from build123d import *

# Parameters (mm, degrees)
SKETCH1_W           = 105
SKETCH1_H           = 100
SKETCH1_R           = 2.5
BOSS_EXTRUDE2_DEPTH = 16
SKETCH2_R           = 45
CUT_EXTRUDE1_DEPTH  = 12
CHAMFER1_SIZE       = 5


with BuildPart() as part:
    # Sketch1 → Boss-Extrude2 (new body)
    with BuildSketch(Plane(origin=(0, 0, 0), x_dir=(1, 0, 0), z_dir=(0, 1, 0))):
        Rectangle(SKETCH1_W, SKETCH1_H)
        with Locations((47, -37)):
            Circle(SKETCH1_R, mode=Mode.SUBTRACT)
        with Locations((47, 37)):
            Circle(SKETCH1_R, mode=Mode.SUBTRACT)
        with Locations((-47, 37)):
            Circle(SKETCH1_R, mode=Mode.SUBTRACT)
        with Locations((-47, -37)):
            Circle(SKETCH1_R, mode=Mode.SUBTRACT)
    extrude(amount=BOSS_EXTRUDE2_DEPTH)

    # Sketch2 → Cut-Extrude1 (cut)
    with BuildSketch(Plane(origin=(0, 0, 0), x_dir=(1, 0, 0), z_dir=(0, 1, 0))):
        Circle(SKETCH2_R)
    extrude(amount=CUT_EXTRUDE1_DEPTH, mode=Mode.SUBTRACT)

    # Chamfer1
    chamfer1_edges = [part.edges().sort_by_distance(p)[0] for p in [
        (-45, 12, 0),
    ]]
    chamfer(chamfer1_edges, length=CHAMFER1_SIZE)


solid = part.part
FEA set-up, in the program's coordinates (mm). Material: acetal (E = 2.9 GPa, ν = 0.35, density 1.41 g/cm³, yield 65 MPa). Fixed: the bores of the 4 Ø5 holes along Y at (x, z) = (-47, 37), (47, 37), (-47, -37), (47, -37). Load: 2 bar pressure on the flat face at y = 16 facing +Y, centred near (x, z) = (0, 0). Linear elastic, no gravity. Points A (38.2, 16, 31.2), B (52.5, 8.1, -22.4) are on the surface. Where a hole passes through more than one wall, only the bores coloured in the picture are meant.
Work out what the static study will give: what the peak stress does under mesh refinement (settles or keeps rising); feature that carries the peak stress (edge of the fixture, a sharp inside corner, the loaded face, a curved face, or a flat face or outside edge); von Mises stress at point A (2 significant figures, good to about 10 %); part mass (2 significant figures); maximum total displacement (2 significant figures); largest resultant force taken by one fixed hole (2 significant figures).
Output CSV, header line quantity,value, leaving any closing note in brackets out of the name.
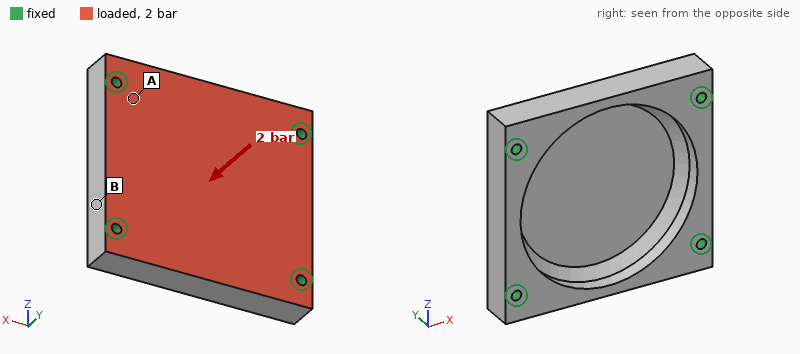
quantity,value
what the peak stress does under mesh refinement,keeps rising
feature that carries the peak stress,edge of the fixture
von Mises stress at point A,3.6 MPa
part mass,130 g
maximum total displacement,0.77 mm
largest resultant force taken by one fixed hole,600 N
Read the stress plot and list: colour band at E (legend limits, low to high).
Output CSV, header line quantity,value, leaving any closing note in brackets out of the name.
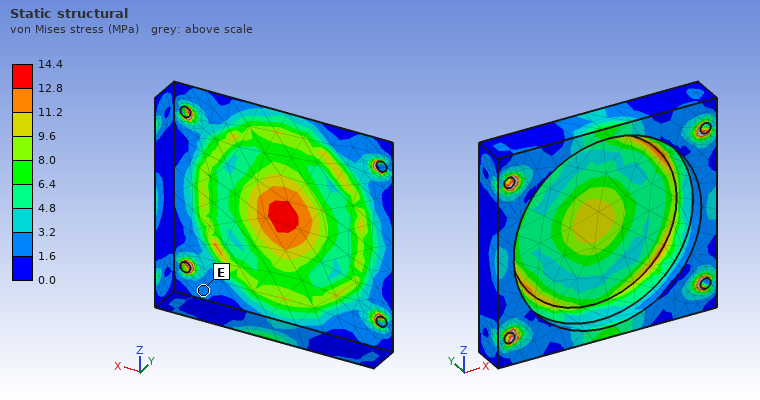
quantity,value
colour band at E,1.6 to 3.2 MPa
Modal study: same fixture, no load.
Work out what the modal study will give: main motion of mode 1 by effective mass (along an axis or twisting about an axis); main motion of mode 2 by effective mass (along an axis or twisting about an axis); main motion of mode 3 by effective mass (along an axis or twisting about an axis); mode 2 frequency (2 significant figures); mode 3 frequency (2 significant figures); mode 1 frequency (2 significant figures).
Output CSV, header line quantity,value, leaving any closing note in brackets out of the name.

quantity,value
main motion of mode 1 by effective mass,along Y
main motion of mode 2 by effective mass,twisting about X
main motion of mode 3 by effective mass,along Y
mode 2 frequency,2200 Hz
mode 3 frequency,2500 Hz
mode 1 frequency,1400 Hz
